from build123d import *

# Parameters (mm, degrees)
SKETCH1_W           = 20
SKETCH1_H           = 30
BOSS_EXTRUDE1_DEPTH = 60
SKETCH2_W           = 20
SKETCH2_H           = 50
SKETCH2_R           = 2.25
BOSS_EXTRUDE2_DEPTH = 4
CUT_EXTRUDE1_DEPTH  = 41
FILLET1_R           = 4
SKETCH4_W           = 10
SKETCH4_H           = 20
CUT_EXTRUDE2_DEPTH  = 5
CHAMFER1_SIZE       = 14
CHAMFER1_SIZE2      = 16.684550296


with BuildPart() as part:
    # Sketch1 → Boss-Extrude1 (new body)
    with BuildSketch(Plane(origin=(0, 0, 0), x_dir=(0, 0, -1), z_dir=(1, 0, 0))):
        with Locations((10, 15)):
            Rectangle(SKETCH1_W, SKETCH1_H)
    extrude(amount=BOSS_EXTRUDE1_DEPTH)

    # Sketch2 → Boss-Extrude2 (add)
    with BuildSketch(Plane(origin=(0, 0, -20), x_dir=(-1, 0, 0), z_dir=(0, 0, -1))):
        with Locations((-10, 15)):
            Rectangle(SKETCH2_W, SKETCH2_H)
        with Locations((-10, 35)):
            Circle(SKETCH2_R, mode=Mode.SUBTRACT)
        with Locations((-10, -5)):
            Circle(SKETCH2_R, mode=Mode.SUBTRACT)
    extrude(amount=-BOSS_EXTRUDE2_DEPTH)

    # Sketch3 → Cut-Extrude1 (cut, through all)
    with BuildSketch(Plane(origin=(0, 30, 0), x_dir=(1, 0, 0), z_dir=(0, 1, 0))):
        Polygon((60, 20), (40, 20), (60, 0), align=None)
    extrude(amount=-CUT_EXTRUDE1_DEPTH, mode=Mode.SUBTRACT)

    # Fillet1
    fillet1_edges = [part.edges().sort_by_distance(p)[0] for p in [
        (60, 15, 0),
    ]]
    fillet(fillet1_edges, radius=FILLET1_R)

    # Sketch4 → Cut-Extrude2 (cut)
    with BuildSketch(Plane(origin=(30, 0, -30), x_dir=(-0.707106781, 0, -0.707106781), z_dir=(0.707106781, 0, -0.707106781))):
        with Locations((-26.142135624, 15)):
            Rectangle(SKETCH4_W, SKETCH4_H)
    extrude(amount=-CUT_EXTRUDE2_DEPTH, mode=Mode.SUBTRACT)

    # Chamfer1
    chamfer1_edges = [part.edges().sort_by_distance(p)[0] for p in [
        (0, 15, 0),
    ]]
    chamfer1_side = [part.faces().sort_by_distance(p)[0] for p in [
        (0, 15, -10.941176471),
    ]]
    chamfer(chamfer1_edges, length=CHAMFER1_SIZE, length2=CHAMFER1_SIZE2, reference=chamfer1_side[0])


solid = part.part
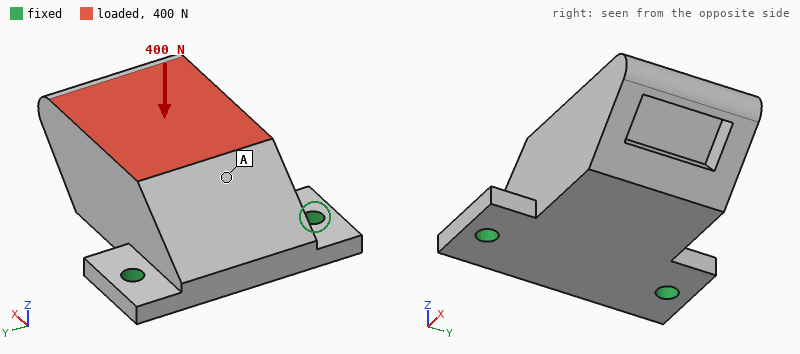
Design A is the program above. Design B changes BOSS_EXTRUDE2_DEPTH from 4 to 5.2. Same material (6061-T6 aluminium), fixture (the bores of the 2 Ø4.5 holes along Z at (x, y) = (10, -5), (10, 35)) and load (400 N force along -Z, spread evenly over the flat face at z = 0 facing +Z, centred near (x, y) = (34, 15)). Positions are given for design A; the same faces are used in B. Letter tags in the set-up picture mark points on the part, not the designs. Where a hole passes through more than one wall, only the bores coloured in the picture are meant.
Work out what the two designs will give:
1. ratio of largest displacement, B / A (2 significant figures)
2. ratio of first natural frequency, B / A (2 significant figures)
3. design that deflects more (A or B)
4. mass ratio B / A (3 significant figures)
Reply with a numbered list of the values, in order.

1. 0.61
2. 1.3
3. A
4. 1.02
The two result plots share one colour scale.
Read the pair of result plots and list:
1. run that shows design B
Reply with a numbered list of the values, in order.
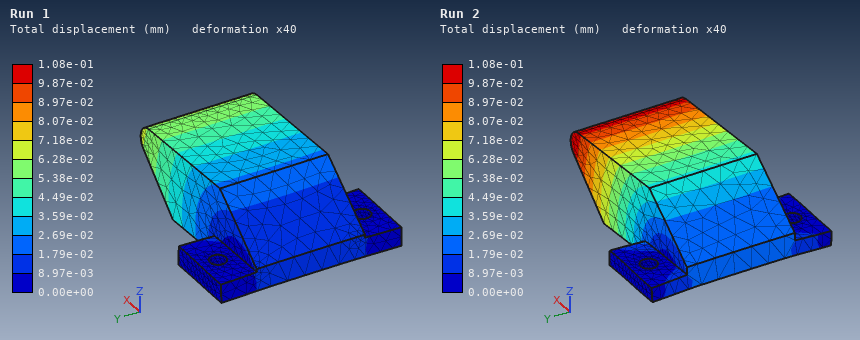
1. Run 1
